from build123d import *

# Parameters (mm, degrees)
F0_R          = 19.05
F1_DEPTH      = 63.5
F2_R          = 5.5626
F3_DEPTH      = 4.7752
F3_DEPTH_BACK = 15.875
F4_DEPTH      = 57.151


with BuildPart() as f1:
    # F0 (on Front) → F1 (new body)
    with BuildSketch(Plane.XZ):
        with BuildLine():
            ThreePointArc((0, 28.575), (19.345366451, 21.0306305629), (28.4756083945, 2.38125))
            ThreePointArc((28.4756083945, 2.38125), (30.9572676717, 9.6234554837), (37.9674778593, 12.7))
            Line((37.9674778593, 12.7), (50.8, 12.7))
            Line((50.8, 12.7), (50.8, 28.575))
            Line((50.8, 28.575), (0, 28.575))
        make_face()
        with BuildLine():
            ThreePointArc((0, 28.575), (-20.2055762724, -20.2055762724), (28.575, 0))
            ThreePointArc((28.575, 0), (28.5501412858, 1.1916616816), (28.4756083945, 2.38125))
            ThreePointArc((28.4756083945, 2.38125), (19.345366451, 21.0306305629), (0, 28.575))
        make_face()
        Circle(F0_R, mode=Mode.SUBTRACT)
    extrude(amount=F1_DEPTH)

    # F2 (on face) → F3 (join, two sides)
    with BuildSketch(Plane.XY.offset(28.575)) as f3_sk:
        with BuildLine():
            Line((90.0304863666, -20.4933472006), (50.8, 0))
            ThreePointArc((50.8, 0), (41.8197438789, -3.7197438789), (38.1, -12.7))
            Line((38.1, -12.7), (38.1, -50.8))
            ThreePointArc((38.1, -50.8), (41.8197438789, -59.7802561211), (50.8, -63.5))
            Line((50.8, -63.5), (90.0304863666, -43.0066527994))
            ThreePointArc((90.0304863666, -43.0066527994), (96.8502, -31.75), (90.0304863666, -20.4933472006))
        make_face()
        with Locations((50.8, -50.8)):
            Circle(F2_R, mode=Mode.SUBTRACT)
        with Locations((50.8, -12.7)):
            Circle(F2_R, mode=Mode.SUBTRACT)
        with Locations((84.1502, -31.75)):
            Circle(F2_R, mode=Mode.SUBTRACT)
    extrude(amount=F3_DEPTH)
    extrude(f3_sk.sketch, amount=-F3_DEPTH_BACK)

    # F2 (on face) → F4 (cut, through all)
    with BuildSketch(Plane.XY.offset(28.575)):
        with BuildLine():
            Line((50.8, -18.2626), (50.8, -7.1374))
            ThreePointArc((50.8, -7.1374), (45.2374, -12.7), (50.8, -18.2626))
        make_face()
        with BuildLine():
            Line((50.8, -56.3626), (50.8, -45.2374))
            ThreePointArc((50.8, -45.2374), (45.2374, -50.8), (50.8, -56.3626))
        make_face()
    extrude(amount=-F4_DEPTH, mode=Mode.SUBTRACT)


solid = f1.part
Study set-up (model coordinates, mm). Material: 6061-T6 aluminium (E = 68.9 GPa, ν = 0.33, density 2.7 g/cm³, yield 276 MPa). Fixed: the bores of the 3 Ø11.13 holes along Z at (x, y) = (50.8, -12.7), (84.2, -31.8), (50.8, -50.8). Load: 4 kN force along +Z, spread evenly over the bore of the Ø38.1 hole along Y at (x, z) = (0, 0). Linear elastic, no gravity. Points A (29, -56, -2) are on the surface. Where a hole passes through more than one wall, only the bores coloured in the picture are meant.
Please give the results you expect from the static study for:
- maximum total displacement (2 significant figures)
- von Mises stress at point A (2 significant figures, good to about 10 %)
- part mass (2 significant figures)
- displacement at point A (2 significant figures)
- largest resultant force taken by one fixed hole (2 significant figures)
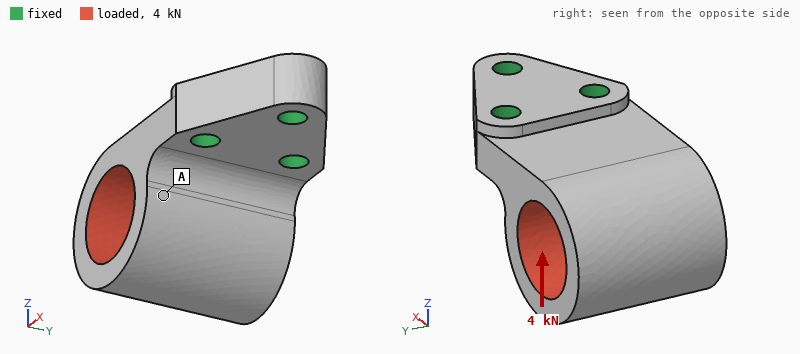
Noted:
0.18 mm
11 MPa
430 g
0.049 mm
2.3 kN
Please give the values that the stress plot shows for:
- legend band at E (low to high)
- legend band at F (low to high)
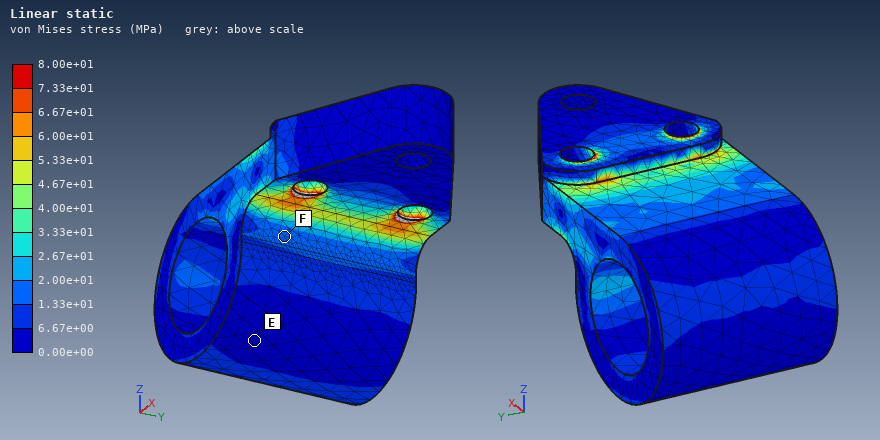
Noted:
0.00e+00 to 6.67e+00 MPa
1.33e+01 to 2.00e+01 MPa
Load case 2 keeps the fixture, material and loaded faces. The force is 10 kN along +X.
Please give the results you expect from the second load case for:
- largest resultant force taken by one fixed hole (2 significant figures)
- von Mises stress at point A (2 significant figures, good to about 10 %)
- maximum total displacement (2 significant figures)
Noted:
4.8 kN
31 MPa
0.27 mm
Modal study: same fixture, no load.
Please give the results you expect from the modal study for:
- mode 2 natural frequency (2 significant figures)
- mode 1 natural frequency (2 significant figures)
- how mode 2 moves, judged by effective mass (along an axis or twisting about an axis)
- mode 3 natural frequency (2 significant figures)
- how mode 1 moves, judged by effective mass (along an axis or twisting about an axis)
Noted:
3700 Hz
1600 Hz
along Y
5900 Hz
along Z
